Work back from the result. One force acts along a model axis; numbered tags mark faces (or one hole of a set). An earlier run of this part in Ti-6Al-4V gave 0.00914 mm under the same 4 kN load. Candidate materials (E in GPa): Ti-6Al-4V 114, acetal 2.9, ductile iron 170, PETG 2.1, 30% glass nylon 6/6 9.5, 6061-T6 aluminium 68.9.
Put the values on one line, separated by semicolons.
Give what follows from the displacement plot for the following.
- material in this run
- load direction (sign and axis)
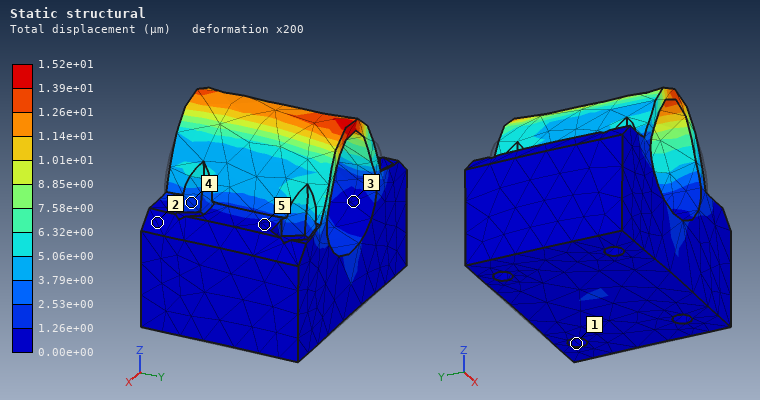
6061-T6 aluminium; +Z
